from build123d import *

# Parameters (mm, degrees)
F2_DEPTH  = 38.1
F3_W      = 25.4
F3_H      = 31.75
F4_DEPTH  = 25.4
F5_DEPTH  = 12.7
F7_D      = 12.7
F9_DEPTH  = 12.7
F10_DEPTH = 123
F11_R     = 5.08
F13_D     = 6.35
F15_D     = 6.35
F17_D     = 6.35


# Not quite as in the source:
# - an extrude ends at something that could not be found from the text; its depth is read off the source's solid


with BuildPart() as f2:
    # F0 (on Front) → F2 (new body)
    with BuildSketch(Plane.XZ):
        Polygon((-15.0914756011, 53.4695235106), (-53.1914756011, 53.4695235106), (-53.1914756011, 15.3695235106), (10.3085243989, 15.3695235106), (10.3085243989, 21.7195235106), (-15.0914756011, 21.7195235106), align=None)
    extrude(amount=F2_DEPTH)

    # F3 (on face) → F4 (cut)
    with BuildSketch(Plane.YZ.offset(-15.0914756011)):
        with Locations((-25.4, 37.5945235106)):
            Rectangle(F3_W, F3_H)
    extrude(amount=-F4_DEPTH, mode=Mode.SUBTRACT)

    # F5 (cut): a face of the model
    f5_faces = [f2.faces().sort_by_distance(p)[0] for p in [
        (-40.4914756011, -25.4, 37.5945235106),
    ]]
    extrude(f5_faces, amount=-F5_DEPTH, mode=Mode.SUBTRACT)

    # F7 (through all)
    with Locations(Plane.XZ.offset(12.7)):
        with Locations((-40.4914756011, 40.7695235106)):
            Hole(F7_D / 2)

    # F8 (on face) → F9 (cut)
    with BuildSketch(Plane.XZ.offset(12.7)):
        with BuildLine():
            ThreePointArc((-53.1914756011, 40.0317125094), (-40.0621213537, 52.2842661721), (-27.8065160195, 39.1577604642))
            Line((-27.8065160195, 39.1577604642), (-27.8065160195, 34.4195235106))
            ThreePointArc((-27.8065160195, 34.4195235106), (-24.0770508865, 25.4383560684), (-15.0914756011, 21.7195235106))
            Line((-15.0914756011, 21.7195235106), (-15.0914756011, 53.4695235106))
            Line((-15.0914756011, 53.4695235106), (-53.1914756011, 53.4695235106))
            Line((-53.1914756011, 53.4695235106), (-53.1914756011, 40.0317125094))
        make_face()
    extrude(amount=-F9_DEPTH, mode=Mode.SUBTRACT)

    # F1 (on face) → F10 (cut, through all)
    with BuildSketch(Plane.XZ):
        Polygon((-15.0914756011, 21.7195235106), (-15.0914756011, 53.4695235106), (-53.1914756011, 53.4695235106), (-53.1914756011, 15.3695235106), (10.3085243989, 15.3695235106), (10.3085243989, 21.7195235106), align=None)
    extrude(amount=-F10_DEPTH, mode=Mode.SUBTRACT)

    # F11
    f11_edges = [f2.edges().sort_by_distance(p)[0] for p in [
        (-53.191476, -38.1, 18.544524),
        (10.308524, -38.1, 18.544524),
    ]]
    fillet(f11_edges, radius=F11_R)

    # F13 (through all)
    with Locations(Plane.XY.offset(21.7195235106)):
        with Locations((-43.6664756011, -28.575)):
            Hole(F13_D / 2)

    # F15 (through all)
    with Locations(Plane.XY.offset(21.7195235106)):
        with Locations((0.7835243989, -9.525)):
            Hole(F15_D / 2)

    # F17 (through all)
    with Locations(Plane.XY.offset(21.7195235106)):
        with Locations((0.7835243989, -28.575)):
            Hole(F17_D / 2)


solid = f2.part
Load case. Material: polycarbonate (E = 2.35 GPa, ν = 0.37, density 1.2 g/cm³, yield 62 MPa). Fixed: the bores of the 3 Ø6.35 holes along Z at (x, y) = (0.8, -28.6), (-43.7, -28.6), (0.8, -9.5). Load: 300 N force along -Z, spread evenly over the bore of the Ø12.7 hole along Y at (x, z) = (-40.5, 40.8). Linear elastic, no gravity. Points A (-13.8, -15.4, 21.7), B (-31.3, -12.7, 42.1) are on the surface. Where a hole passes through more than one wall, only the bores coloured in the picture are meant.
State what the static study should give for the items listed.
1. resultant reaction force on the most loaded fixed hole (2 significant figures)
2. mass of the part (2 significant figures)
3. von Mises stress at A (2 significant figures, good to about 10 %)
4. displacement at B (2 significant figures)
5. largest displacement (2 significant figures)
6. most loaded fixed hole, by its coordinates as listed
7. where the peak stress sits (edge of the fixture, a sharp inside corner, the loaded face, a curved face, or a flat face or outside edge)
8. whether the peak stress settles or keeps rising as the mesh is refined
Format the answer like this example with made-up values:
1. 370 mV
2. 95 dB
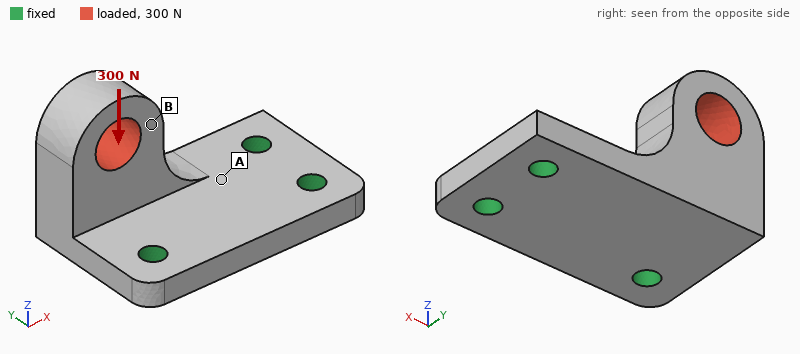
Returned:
1. 240 N
2. 27 g
3. 6.9 MPa
4. 0.56 mm
5. 0.95 mm
6. (-43.7, -28.6)
7. edge of the fixture
8. keeps rising
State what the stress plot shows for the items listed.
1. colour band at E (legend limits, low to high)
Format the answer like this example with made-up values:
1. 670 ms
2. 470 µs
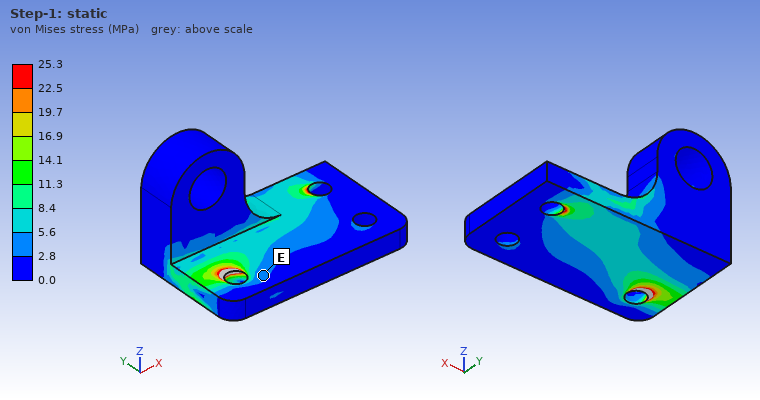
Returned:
1. 2.8 to 5.6 MPa
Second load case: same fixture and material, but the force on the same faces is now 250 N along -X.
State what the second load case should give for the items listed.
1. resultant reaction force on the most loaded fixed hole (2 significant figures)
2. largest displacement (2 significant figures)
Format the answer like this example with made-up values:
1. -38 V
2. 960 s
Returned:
1. 160 N
2. 0.53 mm
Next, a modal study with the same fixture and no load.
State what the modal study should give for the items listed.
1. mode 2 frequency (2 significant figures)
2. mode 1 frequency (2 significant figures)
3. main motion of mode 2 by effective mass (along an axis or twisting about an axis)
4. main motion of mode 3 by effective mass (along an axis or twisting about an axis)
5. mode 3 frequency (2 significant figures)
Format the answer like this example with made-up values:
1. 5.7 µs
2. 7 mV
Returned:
1. 1900 Hz
2. 860 Hz
3. along X
4. along Z
5. 2600 Hz
